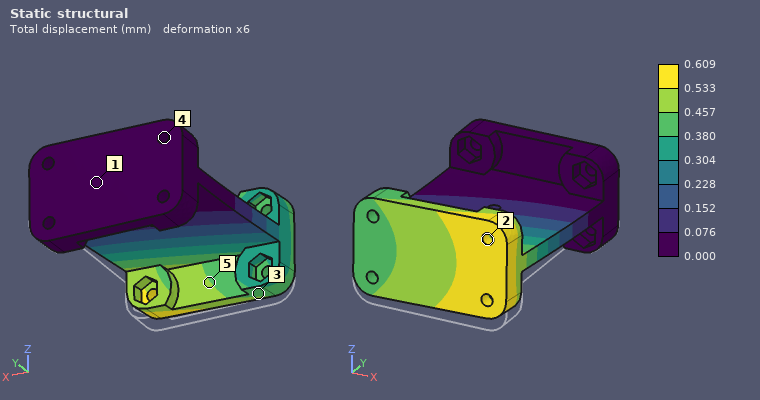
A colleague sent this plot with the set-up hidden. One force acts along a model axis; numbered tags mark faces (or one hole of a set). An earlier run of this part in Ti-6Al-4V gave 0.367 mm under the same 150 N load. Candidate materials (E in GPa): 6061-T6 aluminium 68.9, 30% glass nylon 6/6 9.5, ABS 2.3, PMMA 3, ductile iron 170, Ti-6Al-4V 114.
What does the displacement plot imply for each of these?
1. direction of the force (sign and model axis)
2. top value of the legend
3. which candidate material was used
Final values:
+Z
0.609 mm
6061-T6 aluminium
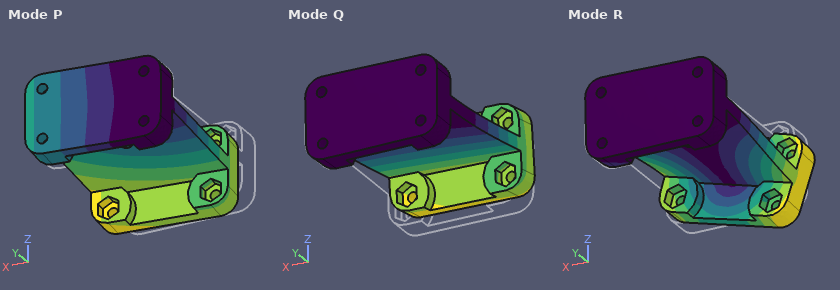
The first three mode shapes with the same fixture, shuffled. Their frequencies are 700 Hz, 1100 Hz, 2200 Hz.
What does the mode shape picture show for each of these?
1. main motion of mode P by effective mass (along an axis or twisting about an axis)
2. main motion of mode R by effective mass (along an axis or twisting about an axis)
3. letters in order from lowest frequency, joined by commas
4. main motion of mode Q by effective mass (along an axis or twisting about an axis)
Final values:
along X
twisting about Y
Q, P, R
along Z
